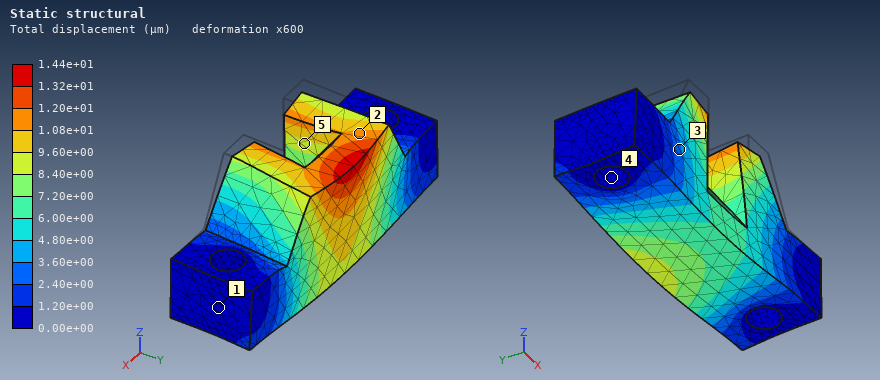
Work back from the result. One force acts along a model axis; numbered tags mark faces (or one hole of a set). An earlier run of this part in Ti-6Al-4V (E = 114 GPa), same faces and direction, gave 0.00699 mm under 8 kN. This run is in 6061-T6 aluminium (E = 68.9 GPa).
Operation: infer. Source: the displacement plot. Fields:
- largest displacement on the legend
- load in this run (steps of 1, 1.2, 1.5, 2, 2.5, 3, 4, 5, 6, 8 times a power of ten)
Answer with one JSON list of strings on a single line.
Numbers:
["1.44e+01 µm", "10 kN"]
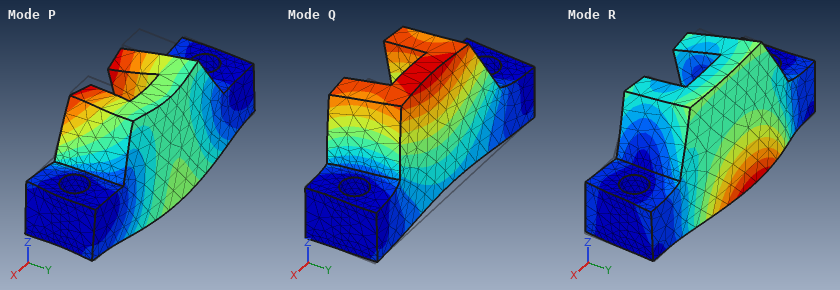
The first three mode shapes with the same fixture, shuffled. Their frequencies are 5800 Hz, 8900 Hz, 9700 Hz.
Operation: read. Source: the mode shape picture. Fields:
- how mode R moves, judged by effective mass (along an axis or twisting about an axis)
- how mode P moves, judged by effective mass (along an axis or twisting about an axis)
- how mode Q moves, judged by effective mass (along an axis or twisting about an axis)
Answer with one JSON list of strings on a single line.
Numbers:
["along Y", "along Z", "along Y"]
